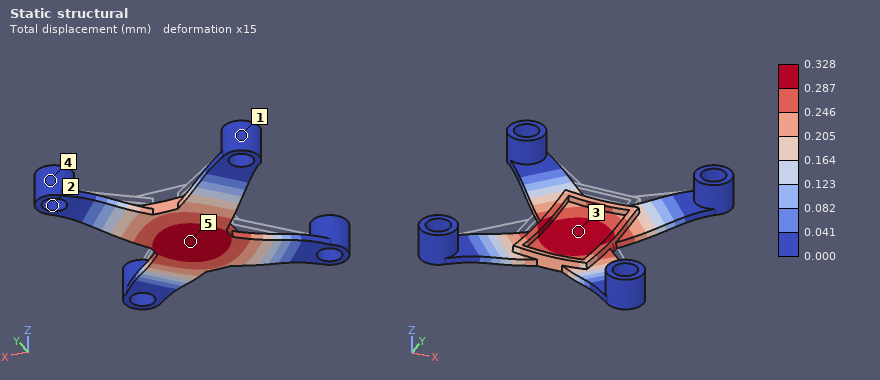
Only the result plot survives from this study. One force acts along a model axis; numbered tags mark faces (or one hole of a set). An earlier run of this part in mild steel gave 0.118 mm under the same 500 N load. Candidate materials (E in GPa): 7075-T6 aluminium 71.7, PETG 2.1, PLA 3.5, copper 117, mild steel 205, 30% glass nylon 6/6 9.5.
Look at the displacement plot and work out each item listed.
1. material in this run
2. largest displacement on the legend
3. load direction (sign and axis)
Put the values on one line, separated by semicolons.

7075-T6 aluminium; 0.328 mm; -Z
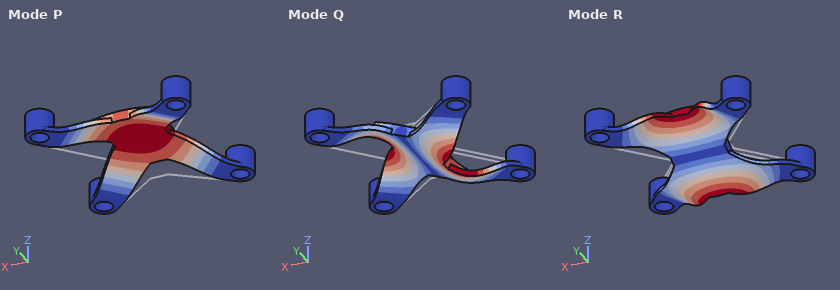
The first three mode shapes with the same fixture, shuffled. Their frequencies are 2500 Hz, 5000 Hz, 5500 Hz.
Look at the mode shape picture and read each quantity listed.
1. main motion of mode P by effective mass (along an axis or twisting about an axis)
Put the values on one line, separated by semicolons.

along Z
